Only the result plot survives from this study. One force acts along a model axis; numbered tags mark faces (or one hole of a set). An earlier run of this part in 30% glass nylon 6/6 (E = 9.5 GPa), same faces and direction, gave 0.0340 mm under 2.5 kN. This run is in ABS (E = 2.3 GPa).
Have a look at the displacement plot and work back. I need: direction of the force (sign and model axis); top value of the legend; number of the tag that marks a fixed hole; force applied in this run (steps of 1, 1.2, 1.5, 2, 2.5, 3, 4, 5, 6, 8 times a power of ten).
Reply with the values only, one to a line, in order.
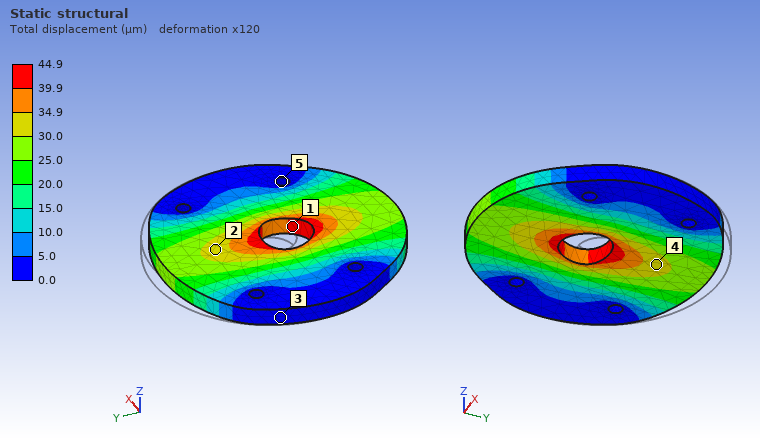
-Y
44.9 µm
5
800 N
